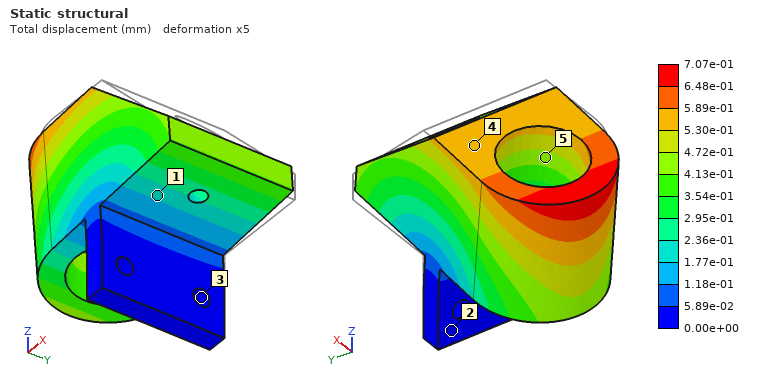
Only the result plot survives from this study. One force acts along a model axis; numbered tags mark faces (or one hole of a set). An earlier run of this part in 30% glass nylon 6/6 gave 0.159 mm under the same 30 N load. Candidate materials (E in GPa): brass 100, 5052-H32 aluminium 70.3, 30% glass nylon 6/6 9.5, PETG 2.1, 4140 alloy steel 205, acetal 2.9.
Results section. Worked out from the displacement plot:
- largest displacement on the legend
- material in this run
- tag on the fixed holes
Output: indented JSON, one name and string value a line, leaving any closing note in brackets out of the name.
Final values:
{
  "largest displacement on the legend": "7.07e-01 mm",
  "material in this run": "PETG",
  "tag on the fixed holes": "3"
}
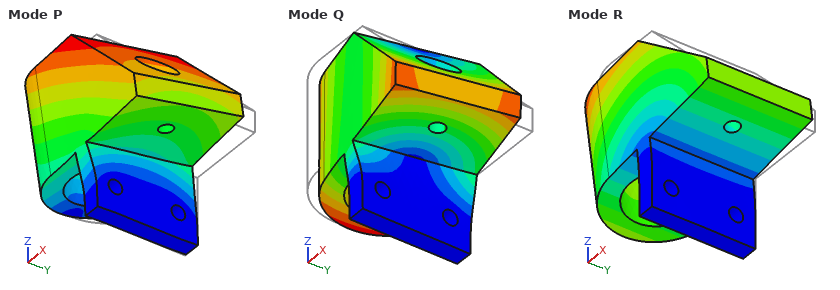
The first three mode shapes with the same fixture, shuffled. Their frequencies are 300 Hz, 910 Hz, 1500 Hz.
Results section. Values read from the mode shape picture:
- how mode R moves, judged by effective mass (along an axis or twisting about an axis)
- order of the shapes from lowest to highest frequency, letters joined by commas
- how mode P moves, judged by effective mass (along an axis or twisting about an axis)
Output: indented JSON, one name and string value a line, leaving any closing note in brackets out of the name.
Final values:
{
  "how mode R moves, judged by effective mass": "along X",
  "order of the shapes from lowest to highest frequency, letters joined by commas": "R, Q, P",
  "how mode P moves, judged by effective mass": "along Y"
}
